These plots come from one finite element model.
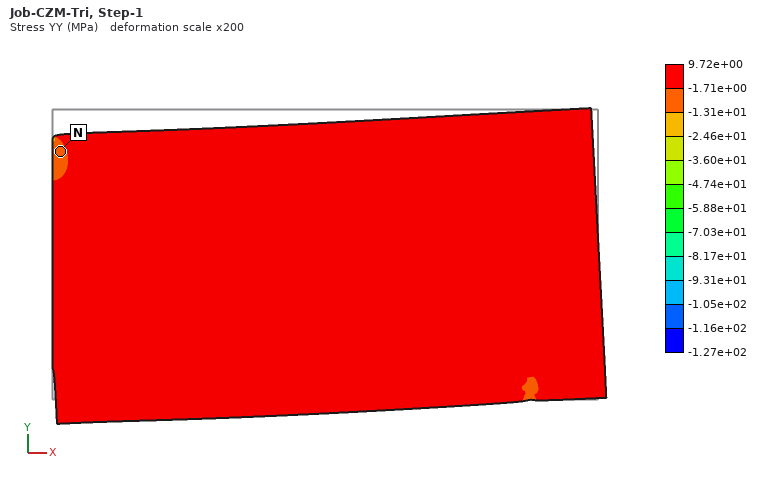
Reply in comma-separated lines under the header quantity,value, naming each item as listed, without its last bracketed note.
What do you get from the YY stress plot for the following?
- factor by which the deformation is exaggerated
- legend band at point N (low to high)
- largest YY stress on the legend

quantity,value
factor by which the deformation is exaggerated,200
legend band at point N,-1.31e+01 to -1.71e+00 MPa
largest YY stress on the legend,9.72e+00 MPa
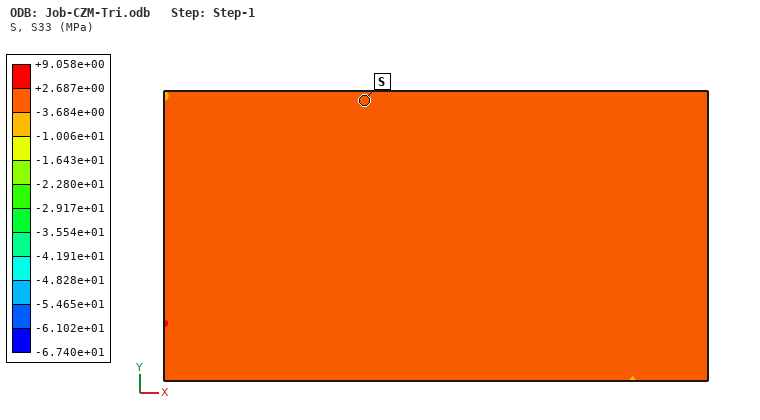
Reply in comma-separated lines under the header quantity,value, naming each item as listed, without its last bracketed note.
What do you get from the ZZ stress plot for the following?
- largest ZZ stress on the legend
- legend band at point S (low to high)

quantity,value
largest ZZ stress on the legend,+9.058e+00 MPa
legend band at point S,-3.684e+00 to +2.687e+00 MPa
